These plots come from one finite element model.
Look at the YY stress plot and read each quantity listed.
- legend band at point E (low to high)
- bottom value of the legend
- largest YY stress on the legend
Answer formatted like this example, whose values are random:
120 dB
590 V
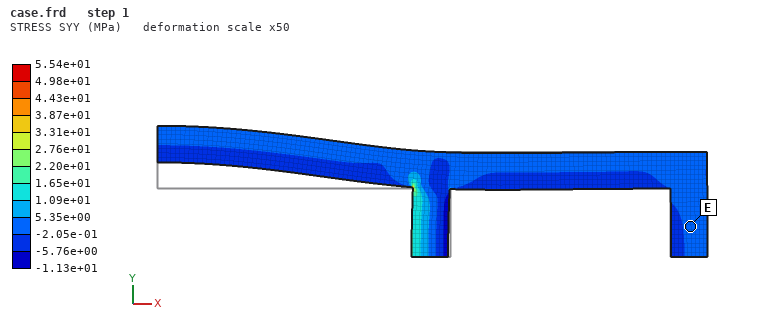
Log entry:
-2.05e-01 to 5.35e+00 MPa
-1.13e+01 MPa
5.54e+01 MPa
